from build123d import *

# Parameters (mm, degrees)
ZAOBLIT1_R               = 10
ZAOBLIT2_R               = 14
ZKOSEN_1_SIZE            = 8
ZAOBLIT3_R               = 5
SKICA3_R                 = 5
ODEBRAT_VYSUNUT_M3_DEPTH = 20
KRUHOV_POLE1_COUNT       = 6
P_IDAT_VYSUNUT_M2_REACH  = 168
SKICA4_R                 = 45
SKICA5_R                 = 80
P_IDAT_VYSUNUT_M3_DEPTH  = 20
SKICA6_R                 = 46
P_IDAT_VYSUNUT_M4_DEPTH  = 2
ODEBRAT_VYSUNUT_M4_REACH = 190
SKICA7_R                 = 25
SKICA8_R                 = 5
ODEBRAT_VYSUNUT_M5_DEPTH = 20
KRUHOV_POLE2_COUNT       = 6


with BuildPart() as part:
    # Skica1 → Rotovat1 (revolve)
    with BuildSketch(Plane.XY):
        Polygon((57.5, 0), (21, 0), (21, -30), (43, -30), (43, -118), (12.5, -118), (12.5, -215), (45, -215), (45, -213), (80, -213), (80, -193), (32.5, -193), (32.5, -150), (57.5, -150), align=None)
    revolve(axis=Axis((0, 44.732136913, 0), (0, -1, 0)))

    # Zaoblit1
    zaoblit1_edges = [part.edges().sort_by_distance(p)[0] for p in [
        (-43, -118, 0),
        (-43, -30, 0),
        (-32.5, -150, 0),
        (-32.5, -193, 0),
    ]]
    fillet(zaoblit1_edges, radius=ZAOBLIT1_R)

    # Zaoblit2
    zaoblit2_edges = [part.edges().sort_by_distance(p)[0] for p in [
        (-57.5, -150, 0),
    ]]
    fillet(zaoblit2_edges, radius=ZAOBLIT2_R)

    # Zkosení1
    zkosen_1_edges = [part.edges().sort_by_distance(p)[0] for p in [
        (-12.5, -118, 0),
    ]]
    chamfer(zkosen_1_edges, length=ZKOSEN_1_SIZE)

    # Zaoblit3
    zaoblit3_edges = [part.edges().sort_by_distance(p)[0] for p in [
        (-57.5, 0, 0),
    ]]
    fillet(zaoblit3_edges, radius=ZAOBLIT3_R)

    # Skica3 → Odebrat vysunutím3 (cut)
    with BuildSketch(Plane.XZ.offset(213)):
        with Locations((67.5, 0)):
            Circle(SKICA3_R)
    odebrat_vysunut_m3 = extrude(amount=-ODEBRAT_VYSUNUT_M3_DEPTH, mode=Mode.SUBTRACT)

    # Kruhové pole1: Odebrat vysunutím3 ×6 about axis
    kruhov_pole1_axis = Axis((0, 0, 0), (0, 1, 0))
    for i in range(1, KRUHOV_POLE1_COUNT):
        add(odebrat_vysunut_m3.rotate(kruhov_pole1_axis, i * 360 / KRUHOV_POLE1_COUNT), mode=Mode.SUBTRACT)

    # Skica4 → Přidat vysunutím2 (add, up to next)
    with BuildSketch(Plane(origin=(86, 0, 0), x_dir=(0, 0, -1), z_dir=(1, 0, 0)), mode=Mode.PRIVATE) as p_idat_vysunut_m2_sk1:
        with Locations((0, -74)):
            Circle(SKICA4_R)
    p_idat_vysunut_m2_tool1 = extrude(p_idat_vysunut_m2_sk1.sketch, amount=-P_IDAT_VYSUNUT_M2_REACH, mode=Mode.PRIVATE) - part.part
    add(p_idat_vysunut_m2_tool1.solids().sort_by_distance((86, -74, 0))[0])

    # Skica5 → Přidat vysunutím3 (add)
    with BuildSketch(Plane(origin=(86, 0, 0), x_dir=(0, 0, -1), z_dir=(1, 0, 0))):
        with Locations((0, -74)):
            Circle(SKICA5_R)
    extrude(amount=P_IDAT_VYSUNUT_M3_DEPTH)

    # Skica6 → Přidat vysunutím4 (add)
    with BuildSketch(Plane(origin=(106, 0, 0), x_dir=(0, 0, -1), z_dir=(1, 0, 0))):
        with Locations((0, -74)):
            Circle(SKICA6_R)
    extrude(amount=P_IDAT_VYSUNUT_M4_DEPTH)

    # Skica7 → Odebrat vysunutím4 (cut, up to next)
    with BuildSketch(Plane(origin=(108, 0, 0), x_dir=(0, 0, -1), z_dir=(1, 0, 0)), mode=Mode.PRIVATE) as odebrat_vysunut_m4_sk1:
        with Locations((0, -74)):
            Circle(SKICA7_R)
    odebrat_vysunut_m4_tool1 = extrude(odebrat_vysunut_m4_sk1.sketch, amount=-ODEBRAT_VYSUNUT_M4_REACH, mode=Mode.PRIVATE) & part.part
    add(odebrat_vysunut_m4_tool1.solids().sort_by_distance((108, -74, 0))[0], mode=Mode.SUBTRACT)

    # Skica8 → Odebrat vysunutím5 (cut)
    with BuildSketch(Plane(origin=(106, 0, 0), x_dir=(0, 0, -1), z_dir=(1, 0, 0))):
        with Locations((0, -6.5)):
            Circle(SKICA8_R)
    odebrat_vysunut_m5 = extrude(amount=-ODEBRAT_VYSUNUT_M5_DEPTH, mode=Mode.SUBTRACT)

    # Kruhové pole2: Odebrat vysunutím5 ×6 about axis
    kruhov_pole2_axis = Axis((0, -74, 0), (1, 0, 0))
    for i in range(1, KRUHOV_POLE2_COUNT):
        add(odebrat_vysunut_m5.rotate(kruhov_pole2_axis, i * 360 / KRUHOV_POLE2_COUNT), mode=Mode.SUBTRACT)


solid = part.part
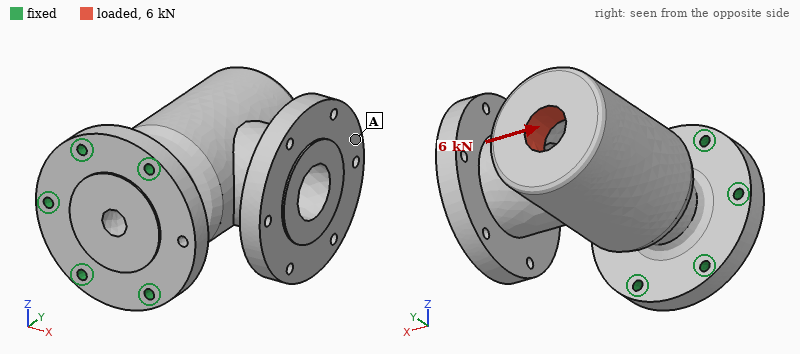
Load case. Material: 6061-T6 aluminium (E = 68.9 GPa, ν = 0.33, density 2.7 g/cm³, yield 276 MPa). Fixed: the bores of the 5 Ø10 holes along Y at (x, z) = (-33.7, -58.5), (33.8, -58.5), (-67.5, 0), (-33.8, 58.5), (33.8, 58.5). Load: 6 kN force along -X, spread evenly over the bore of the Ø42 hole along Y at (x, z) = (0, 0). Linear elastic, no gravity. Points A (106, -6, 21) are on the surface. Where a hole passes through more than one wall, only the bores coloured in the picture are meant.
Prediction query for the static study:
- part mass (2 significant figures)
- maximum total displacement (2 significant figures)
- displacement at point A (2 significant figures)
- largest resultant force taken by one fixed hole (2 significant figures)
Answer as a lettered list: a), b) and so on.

a) 5.4 kg
b) 0.39 mm
c) 0.37 mm
d) 7.5 kN
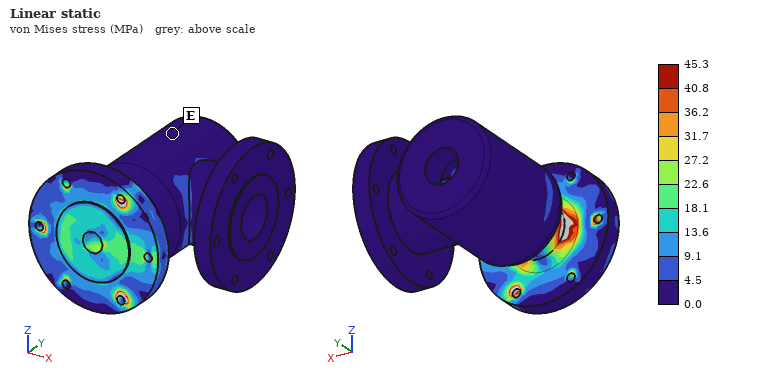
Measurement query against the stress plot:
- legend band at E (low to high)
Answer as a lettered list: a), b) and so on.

a) 0.0 to 4.5 MPa
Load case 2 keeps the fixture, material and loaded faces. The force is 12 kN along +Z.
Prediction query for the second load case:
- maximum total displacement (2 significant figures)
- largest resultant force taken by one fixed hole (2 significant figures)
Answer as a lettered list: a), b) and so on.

a) 0.59 mm
b) 12 kN
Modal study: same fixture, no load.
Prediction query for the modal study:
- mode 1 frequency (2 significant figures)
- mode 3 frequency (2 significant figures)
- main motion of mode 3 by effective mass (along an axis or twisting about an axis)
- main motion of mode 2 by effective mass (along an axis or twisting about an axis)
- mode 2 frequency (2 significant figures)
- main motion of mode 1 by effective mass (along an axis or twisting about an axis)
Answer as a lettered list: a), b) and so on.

a) 460 Hz
b) 1100 Hz
c) twisting about Y
d) along Z
e) 520 Hz
f) along X
